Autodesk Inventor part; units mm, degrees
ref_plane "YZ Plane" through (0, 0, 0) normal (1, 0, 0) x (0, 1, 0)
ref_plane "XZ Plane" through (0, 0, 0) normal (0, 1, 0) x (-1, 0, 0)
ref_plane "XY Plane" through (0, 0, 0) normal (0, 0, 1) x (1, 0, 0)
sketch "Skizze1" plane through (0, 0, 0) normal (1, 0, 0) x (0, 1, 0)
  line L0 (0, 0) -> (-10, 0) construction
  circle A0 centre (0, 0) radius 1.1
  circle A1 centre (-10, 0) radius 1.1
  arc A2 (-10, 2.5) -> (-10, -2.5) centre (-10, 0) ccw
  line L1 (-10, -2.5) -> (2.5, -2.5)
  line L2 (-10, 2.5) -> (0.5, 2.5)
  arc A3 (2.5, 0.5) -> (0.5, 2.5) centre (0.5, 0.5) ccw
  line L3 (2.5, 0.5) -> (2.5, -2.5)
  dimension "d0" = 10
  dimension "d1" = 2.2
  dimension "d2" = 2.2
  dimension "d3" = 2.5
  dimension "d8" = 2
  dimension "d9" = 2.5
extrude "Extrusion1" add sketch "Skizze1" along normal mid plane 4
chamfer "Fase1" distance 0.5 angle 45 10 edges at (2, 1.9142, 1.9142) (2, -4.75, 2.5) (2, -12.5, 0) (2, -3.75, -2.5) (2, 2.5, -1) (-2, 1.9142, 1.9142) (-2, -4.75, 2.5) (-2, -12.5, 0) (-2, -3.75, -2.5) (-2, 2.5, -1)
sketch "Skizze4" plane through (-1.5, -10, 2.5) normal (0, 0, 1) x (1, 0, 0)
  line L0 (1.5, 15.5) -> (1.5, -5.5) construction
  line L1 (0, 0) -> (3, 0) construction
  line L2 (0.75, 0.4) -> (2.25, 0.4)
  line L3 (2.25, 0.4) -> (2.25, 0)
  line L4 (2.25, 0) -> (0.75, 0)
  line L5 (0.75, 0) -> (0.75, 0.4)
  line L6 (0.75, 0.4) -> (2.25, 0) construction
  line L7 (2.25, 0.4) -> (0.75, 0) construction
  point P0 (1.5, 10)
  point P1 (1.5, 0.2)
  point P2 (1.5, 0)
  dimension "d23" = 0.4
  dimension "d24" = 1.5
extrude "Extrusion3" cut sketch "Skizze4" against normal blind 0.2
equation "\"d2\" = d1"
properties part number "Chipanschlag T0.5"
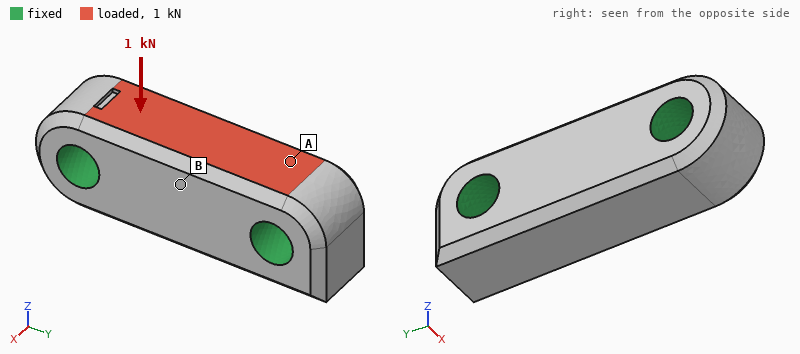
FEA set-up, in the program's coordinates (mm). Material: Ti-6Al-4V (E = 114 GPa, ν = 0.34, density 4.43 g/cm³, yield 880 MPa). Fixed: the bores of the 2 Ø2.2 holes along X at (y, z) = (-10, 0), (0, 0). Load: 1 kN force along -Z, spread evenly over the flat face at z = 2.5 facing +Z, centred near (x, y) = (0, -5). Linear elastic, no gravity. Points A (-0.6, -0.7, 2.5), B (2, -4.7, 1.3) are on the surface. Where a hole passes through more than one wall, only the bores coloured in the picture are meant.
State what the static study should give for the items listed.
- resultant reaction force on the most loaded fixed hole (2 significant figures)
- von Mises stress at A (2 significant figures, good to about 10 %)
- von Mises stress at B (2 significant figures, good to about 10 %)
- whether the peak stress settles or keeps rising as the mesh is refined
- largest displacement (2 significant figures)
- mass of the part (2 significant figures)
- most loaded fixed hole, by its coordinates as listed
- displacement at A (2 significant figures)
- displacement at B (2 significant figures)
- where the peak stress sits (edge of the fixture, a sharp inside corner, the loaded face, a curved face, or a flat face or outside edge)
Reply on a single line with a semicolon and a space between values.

540 N; 35 MPa; 13 MPa; keeps rising; 2.2 µm; 1.1 g; (0, 0); 0.82 µm; 2.0 µm; edge of the fixture
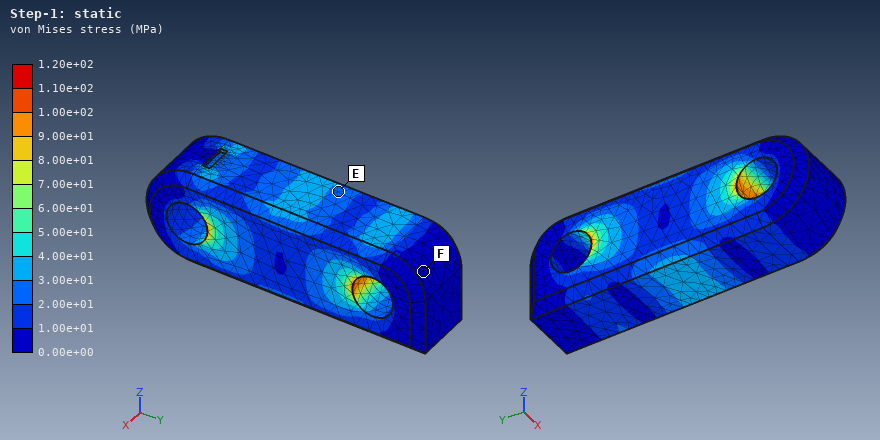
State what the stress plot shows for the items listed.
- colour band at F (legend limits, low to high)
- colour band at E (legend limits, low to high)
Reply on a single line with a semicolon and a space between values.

0.00e+00 to 1.00e+01 MPa; 2.00e+01 to 3.00e+01 MPa
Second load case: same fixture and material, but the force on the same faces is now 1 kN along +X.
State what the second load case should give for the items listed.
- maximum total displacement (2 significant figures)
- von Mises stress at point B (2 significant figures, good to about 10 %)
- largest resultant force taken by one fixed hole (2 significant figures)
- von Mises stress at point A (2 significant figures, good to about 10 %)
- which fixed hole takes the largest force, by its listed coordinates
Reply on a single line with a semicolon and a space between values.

5.7 µm; 50 MPa; 530 N; 87 MPa; (0, 0)
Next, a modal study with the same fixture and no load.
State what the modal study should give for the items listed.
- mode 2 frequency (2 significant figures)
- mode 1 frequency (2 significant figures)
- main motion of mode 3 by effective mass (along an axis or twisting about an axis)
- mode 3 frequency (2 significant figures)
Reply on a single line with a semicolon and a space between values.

140 kHz; 140 kHz; twisting about Y; 160 kHz
